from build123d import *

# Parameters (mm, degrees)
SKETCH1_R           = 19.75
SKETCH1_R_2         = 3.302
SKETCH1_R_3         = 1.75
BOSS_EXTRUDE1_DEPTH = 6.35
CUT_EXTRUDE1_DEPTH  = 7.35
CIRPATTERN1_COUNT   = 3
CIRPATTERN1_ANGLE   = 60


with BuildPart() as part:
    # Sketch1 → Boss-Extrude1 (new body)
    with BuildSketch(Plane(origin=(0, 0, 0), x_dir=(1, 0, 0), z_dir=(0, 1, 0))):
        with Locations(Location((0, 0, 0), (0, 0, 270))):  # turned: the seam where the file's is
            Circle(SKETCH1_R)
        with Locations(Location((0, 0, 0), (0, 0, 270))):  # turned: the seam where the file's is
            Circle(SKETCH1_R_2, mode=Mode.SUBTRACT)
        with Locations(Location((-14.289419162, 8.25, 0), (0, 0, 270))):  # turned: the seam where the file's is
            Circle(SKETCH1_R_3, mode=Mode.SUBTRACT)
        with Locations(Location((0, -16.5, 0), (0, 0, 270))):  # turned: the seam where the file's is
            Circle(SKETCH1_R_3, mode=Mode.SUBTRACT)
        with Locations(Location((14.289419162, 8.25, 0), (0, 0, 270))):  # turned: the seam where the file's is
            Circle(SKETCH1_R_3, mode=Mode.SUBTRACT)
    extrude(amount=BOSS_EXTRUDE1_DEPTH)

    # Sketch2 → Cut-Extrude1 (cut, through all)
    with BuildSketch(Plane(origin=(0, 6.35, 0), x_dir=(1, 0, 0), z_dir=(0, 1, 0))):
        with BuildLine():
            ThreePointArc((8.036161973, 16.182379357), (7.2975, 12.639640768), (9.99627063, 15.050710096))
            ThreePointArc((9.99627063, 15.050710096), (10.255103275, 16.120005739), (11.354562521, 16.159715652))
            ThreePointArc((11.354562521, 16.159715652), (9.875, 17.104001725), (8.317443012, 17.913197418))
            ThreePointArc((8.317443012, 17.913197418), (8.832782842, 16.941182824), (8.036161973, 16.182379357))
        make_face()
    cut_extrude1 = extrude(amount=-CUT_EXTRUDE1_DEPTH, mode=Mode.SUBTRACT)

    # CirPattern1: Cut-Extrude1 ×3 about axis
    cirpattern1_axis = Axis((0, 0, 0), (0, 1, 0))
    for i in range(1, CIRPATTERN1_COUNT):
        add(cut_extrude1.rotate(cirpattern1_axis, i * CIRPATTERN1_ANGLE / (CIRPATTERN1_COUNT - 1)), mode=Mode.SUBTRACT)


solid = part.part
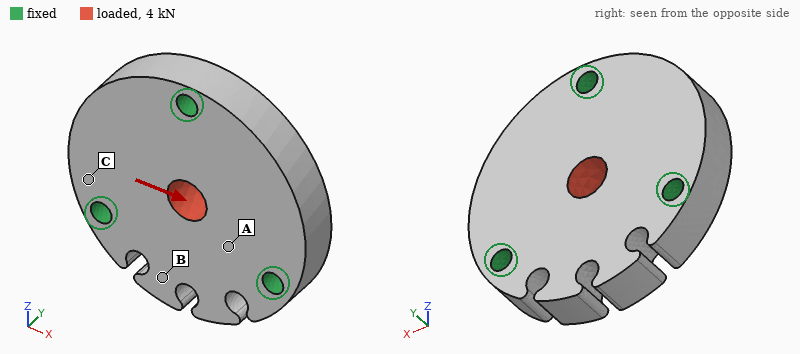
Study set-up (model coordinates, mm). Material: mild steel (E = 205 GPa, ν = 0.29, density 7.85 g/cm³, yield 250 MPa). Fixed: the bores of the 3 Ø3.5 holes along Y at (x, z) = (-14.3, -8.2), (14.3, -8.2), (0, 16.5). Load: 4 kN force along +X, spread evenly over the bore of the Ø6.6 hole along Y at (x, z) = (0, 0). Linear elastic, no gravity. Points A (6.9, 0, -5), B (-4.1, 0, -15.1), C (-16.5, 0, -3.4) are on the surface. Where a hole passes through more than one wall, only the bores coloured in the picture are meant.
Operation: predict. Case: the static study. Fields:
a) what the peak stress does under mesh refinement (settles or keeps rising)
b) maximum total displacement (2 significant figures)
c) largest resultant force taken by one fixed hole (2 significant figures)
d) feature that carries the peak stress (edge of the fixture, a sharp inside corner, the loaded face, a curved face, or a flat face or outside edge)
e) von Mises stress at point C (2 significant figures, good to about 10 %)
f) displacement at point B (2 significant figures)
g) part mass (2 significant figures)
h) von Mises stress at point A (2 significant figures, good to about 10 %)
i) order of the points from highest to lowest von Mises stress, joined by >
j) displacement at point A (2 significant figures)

keeps rising
2.3 µm
1.4 kN
edge of the fixture
13 MPa
0.51 µm
56 g
26 MPa
A > C > B
0.95 µm
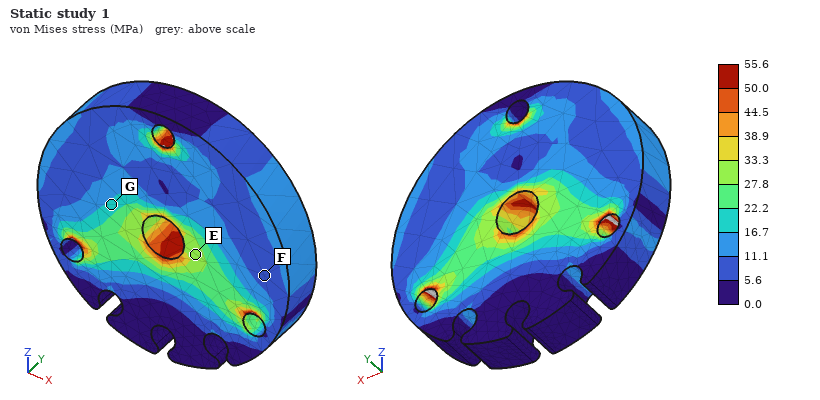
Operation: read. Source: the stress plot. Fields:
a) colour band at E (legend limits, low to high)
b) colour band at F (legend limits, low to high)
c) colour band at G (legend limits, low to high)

27.8 to 33.3 MPa
5.6 to 11.1 MPa
16.7 to 22.2 MPa
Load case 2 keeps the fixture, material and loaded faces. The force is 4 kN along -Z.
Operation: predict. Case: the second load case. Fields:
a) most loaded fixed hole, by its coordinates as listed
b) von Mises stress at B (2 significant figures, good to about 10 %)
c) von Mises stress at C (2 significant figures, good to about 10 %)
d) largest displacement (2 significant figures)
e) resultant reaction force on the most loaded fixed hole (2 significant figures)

(0, 16.5)
5.5 MPa
11 MPa
2.8 µm
1.6 kN
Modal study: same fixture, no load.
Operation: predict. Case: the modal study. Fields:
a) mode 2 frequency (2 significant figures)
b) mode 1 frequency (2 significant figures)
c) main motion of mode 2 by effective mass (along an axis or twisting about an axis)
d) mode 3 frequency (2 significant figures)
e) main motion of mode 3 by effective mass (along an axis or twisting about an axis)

24 kHz
22 kHz
twisting about Z
26 kHz
along Y
